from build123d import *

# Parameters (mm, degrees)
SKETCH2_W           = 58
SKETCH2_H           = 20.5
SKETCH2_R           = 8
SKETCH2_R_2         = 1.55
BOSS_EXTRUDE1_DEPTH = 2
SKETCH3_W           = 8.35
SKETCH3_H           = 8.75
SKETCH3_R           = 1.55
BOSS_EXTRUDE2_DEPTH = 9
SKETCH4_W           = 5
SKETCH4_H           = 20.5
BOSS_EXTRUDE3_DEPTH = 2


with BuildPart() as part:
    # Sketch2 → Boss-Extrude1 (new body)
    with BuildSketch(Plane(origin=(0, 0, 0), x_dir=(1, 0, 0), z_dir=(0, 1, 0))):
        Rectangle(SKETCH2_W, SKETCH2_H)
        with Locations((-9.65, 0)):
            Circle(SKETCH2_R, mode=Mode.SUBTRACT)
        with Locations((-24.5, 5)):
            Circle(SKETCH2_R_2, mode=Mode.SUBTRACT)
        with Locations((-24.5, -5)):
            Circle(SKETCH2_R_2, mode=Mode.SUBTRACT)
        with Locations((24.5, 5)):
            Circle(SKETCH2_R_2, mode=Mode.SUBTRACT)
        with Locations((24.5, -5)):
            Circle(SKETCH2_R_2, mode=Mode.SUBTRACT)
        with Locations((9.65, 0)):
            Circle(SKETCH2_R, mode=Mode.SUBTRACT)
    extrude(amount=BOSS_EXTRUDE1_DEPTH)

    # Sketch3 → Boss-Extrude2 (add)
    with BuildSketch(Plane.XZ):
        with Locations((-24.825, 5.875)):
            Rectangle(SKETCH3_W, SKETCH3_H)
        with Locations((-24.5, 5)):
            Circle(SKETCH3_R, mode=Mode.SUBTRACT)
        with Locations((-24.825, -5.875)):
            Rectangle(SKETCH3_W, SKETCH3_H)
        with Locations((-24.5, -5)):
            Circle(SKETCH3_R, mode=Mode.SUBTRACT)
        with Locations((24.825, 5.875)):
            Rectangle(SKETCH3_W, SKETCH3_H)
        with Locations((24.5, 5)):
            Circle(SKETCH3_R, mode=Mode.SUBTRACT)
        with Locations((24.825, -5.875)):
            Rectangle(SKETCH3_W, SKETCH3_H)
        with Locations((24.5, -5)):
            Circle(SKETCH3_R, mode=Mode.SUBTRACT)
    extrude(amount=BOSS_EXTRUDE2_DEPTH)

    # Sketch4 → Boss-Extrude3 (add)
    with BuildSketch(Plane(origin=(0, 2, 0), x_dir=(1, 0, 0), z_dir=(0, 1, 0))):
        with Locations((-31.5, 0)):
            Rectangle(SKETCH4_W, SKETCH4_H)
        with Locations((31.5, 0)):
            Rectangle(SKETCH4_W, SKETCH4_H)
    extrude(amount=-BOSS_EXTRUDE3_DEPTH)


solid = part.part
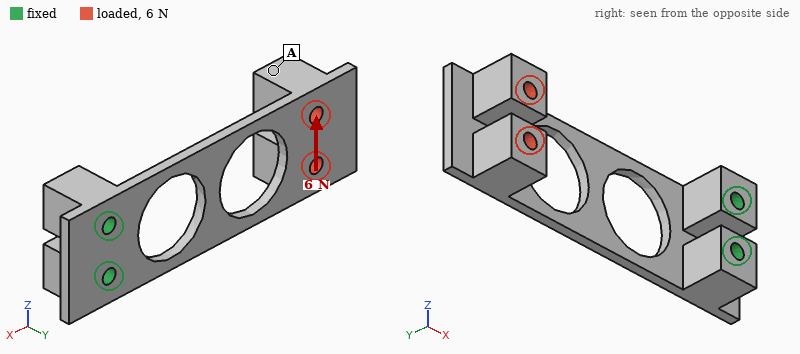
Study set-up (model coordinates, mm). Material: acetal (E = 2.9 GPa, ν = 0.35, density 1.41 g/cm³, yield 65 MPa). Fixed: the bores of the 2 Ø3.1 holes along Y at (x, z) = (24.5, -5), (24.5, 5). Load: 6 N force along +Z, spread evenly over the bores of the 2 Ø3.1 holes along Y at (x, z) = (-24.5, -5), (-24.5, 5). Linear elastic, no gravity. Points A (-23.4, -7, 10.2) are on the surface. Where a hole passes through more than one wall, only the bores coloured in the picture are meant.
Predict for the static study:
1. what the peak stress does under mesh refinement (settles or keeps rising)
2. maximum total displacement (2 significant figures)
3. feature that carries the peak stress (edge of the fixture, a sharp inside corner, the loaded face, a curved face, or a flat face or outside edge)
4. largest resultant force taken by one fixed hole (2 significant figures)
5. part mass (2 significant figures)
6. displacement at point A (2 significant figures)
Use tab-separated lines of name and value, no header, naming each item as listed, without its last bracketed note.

what the peak stress does under mesh refinement	keeps rising
maximum total displacement	0.75 mm
feature that carries the peak stress	a sharp inside corner
largest resultant force taken by one fixed hole	20 N
part mass	6.0 g
displacement at point A	0.66 mm
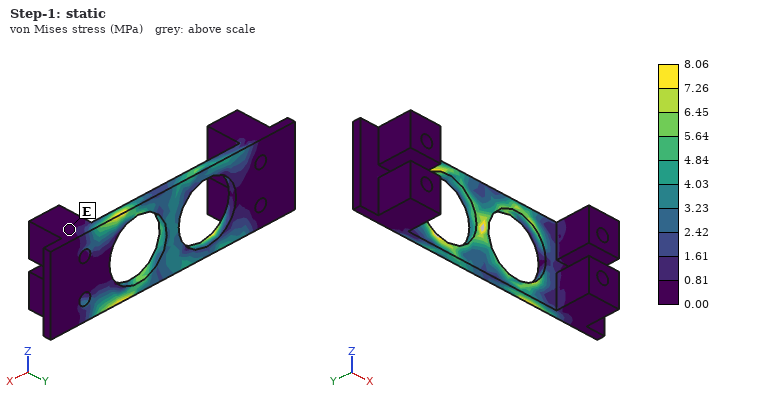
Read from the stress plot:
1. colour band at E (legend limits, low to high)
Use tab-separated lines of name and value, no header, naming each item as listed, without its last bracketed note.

colour band at E	0.00 to 0.81 MPa
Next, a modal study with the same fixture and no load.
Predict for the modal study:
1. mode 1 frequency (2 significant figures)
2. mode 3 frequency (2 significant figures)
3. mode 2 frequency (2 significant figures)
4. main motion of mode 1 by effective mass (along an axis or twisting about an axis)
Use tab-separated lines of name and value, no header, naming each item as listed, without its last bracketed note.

mode 1 frequency	63 Hz
mode 3 frequency	580 Hz
mode 2 frequency	290 Hz
main motion of mode 1 by effective mass	along Y
